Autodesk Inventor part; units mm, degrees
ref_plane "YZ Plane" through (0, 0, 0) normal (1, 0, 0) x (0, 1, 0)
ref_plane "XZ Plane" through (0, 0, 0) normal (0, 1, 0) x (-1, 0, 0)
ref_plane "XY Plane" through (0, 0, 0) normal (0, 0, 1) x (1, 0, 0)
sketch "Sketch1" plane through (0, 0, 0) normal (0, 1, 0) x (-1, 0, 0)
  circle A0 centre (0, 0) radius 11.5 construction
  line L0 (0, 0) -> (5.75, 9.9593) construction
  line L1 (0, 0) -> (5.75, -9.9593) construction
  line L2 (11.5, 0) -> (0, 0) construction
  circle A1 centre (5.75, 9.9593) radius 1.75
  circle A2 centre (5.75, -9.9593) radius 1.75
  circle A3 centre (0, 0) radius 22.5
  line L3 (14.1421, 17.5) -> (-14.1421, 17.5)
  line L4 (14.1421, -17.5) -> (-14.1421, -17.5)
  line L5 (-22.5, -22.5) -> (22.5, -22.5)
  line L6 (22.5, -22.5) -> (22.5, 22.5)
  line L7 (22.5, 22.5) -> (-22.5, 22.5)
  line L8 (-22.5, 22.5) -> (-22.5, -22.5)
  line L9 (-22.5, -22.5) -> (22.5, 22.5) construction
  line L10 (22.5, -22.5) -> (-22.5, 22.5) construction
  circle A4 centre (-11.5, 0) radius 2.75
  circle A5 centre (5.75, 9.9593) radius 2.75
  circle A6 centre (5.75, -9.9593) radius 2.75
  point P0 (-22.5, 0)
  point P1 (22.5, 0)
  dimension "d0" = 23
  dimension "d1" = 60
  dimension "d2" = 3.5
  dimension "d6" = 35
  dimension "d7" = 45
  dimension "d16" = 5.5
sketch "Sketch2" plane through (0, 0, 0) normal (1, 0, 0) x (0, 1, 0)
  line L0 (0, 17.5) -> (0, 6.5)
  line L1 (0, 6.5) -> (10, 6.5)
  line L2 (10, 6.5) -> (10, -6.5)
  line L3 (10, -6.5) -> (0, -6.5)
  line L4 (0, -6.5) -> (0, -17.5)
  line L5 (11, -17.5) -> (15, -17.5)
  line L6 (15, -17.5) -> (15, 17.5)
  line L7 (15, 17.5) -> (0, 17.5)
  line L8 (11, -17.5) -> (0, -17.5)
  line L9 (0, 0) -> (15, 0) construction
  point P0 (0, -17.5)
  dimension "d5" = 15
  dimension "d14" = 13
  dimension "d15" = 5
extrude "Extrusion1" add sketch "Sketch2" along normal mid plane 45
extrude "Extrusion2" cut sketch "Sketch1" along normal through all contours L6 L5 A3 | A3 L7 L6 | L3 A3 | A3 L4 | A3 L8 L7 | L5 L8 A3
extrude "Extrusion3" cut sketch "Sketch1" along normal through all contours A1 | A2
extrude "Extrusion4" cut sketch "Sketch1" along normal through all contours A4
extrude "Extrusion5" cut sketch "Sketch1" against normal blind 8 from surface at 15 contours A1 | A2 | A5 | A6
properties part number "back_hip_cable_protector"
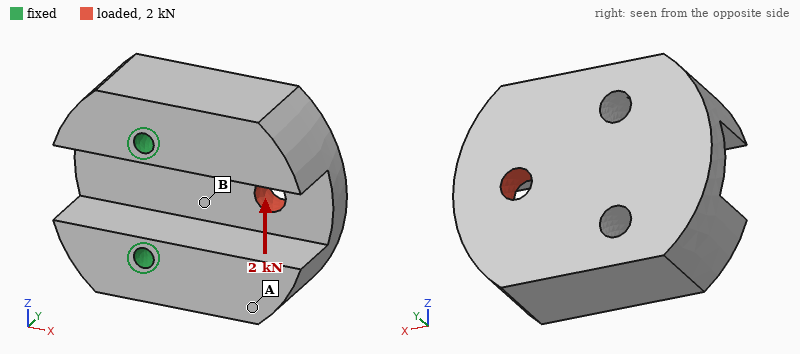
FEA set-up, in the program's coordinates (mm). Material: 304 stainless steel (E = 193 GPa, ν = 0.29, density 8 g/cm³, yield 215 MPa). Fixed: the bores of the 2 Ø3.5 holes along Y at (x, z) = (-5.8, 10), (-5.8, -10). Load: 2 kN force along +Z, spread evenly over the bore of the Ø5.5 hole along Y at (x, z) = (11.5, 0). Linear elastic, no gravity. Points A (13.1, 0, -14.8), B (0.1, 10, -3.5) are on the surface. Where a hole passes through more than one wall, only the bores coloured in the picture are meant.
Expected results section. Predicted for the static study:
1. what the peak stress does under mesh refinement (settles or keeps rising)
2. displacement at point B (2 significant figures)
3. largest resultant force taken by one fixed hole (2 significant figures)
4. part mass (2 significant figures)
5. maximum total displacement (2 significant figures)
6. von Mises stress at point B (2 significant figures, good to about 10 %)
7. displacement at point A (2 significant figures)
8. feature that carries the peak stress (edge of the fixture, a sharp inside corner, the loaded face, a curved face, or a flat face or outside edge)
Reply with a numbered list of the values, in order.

1. keeps rising
2. 3.8 µm
3. 1.7 kN
4. 120 g
5. 10 µm
6. 29 MPa
7. 6.6 µm
8. edge of the fixture
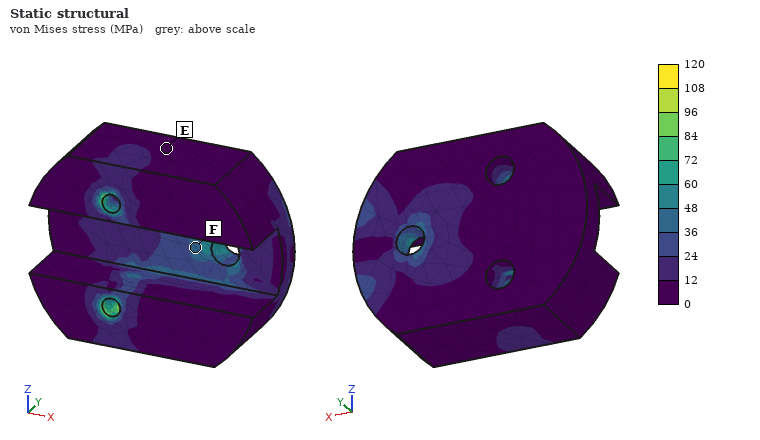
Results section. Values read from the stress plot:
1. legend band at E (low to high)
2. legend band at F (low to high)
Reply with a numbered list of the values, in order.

1. 0 to 12 MPa
2. 36 to 48 MPa
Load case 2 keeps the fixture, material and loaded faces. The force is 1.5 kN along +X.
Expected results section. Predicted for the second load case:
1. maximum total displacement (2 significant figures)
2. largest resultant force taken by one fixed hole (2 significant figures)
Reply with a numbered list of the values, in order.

1. 9.4 µm
2. 750 N
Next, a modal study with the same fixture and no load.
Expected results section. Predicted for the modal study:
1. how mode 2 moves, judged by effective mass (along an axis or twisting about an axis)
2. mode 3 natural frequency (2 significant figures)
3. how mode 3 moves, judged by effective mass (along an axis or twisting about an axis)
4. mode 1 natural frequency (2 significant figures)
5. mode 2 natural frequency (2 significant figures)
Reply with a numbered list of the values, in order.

1. along Z
2. 15 kHz
3. along Z
4. 7200 Hz
5. 9600 Hz
